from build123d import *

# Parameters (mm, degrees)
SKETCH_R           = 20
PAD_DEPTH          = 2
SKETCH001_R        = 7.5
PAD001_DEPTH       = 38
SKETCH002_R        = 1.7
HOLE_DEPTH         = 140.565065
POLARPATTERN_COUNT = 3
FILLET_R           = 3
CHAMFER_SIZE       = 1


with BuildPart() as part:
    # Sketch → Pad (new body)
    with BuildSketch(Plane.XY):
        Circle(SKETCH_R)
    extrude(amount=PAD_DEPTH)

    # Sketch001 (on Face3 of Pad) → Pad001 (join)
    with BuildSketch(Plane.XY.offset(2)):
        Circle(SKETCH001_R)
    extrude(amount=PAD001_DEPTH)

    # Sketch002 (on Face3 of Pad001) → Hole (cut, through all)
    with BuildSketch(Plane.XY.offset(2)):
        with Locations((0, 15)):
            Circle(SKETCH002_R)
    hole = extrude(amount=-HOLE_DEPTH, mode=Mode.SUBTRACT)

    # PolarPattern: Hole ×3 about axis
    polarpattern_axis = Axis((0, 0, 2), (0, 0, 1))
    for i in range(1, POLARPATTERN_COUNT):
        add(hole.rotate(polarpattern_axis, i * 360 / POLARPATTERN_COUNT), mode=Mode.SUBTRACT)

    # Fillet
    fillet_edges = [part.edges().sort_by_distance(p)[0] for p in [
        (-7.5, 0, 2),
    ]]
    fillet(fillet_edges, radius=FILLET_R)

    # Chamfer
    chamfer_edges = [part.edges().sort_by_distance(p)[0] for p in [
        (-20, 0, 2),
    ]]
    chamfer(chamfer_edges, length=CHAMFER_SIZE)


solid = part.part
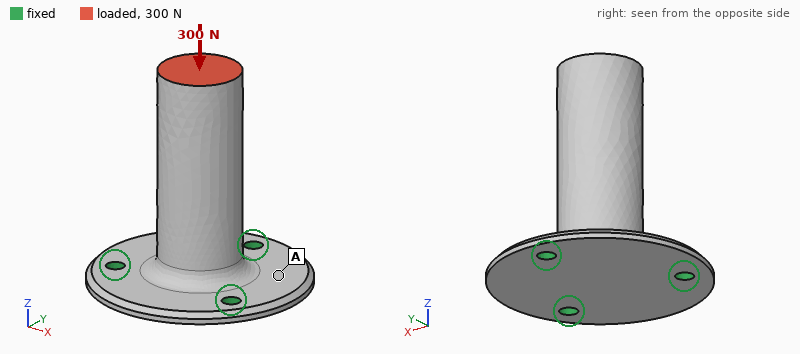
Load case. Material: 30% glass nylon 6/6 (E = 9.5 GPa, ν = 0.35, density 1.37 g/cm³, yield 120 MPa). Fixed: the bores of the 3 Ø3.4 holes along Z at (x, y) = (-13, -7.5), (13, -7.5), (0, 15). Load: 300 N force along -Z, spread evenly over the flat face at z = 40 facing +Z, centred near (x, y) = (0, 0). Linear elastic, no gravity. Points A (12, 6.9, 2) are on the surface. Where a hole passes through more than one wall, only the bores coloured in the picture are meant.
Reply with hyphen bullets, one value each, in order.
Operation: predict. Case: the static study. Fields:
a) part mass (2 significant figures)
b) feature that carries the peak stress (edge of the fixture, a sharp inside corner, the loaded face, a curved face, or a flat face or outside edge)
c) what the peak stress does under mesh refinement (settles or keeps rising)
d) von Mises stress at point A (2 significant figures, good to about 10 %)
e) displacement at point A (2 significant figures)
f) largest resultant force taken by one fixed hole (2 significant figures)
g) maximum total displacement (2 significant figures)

- 13 g
- edge of the fixture
- keeps rising
- 5.4 MPa
- 34 µm
- 110 N
- 46 µm
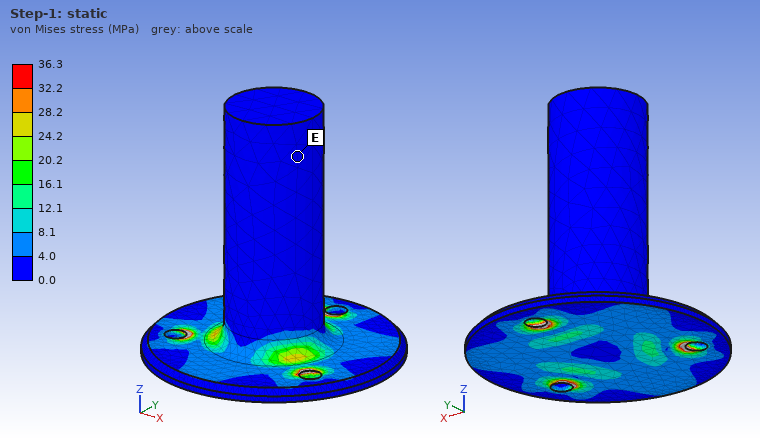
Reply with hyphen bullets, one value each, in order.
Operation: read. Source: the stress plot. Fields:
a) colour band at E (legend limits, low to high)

- 0.0 to 4.0 MPa
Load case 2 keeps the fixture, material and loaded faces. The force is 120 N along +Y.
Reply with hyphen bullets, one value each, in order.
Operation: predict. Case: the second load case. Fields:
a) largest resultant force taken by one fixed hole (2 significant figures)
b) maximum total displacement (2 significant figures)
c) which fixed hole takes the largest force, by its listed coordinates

- 250 N
- 0.43 mm
- (0, 15)
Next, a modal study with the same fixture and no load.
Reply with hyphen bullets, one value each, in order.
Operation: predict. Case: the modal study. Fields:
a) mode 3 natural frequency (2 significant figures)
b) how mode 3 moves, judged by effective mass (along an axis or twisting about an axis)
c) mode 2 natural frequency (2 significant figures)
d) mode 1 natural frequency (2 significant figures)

- 4100 Hz
- along Z
- 1500 Hz
- 1500 Hz
